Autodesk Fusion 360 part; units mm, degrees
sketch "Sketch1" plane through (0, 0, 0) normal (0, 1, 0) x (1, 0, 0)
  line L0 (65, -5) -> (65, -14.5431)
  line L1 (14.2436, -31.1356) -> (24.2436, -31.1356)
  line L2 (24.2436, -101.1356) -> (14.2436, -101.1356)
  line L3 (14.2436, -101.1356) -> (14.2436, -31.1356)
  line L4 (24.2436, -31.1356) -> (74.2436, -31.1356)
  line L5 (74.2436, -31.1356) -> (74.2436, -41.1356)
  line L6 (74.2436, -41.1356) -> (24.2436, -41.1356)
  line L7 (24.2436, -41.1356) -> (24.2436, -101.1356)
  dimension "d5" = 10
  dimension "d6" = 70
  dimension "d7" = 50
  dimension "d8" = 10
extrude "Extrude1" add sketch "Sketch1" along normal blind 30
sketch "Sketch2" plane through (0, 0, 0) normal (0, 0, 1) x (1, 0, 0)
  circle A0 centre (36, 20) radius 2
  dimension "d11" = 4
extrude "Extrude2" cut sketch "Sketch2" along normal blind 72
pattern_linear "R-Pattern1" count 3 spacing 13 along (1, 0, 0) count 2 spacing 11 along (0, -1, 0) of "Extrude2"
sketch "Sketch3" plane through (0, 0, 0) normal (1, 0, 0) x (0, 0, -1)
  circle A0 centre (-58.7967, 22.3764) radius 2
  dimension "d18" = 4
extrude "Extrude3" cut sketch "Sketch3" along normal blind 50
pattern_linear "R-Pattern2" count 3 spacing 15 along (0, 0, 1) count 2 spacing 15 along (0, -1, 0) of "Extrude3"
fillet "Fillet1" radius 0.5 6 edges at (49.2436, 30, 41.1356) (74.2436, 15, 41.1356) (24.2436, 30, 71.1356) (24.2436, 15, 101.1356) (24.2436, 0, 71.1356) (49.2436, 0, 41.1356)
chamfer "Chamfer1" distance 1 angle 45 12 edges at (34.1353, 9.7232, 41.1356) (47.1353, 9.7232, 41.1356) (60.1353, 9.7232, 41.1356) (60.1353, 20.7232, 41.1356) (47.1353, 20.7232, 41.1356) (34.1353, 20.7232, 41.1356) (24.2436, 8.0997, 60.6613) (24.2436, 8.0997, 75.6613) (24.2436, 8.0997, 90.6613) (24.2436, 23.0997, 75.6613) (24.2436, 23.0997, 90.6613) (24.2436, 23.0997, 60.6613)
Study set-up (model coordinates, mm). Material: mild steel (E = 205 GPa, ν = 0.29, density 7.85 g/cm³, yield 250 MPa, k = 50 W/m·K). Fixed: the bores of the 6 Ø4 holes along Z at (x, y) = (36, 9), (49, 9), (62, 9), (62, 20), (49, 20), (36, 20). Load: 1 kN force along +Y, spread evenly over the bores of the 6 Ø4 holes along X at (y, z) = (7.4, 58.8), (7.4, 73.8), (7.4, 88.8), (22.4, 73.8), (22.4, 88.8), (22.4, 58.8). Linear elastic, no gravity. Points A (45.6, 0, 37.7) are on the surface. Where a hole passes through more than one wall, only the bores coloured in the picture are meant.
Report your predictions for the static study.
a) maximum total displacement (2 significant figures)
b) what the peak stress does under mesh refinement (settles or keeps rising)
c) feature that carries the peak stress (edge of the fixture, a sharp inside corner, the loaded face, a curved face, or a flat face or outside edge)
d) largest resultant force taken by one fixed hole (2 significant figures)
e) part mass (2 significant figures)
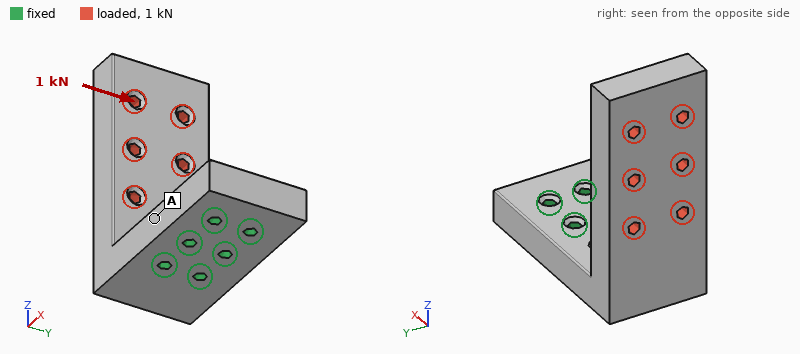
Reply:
51 µm
keeps rising
edge of the fixture
2.0 kN
270 g
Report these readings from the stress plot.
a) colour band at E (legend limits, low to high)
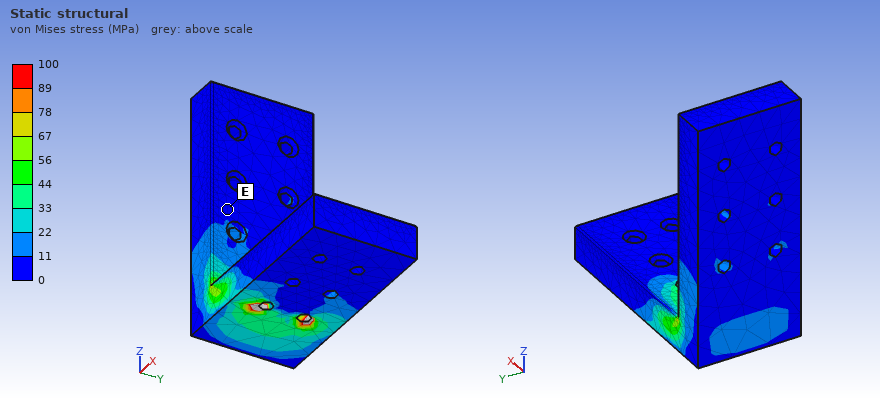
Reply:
0 to 11 MPa
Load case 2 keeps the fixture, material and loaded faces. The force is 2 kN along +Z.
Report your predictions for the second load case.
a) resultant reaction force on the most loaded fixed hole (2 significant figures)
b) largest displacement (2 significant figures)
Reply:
1.3 kN
47 µm
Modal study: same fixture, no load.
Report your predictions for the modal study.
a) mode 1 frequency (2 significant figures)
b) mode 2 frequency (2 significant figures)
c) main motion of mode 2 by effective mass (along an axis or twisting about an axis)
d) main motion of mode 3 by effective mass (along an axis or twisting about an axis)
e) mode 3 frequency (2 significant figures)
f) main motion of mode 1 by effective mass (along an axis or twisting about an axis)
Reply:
1400 Hz
2400 Hz
along Y
along Z
6700 Hz
along X
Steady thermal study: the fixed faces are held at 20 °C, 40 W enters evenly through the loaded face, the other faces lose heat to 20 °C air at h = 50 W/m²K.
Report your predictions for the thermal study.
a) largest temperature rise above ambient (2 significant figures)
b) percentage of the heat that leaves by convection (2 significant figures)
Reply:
83 K
44 %
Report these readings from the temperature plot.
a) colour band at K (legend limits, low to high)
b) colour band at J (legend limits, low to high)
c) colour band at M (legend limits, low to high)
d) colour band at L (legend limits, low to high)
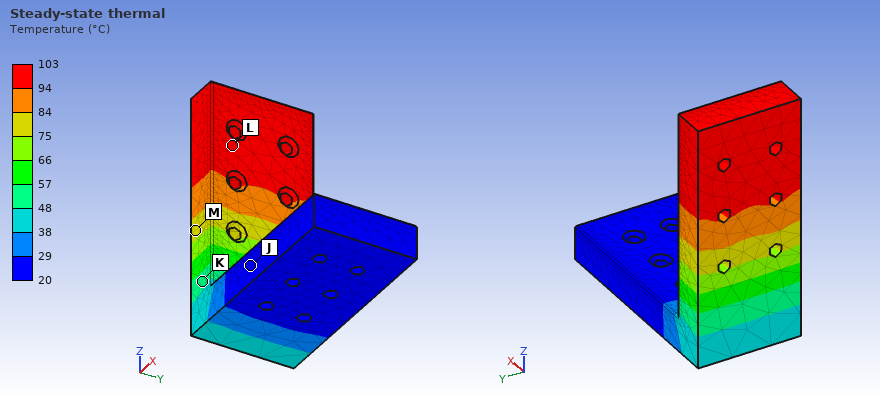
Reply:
48 to 57 °C
20 to 29 °C
75 to 84 °C
94 to 103 °C
